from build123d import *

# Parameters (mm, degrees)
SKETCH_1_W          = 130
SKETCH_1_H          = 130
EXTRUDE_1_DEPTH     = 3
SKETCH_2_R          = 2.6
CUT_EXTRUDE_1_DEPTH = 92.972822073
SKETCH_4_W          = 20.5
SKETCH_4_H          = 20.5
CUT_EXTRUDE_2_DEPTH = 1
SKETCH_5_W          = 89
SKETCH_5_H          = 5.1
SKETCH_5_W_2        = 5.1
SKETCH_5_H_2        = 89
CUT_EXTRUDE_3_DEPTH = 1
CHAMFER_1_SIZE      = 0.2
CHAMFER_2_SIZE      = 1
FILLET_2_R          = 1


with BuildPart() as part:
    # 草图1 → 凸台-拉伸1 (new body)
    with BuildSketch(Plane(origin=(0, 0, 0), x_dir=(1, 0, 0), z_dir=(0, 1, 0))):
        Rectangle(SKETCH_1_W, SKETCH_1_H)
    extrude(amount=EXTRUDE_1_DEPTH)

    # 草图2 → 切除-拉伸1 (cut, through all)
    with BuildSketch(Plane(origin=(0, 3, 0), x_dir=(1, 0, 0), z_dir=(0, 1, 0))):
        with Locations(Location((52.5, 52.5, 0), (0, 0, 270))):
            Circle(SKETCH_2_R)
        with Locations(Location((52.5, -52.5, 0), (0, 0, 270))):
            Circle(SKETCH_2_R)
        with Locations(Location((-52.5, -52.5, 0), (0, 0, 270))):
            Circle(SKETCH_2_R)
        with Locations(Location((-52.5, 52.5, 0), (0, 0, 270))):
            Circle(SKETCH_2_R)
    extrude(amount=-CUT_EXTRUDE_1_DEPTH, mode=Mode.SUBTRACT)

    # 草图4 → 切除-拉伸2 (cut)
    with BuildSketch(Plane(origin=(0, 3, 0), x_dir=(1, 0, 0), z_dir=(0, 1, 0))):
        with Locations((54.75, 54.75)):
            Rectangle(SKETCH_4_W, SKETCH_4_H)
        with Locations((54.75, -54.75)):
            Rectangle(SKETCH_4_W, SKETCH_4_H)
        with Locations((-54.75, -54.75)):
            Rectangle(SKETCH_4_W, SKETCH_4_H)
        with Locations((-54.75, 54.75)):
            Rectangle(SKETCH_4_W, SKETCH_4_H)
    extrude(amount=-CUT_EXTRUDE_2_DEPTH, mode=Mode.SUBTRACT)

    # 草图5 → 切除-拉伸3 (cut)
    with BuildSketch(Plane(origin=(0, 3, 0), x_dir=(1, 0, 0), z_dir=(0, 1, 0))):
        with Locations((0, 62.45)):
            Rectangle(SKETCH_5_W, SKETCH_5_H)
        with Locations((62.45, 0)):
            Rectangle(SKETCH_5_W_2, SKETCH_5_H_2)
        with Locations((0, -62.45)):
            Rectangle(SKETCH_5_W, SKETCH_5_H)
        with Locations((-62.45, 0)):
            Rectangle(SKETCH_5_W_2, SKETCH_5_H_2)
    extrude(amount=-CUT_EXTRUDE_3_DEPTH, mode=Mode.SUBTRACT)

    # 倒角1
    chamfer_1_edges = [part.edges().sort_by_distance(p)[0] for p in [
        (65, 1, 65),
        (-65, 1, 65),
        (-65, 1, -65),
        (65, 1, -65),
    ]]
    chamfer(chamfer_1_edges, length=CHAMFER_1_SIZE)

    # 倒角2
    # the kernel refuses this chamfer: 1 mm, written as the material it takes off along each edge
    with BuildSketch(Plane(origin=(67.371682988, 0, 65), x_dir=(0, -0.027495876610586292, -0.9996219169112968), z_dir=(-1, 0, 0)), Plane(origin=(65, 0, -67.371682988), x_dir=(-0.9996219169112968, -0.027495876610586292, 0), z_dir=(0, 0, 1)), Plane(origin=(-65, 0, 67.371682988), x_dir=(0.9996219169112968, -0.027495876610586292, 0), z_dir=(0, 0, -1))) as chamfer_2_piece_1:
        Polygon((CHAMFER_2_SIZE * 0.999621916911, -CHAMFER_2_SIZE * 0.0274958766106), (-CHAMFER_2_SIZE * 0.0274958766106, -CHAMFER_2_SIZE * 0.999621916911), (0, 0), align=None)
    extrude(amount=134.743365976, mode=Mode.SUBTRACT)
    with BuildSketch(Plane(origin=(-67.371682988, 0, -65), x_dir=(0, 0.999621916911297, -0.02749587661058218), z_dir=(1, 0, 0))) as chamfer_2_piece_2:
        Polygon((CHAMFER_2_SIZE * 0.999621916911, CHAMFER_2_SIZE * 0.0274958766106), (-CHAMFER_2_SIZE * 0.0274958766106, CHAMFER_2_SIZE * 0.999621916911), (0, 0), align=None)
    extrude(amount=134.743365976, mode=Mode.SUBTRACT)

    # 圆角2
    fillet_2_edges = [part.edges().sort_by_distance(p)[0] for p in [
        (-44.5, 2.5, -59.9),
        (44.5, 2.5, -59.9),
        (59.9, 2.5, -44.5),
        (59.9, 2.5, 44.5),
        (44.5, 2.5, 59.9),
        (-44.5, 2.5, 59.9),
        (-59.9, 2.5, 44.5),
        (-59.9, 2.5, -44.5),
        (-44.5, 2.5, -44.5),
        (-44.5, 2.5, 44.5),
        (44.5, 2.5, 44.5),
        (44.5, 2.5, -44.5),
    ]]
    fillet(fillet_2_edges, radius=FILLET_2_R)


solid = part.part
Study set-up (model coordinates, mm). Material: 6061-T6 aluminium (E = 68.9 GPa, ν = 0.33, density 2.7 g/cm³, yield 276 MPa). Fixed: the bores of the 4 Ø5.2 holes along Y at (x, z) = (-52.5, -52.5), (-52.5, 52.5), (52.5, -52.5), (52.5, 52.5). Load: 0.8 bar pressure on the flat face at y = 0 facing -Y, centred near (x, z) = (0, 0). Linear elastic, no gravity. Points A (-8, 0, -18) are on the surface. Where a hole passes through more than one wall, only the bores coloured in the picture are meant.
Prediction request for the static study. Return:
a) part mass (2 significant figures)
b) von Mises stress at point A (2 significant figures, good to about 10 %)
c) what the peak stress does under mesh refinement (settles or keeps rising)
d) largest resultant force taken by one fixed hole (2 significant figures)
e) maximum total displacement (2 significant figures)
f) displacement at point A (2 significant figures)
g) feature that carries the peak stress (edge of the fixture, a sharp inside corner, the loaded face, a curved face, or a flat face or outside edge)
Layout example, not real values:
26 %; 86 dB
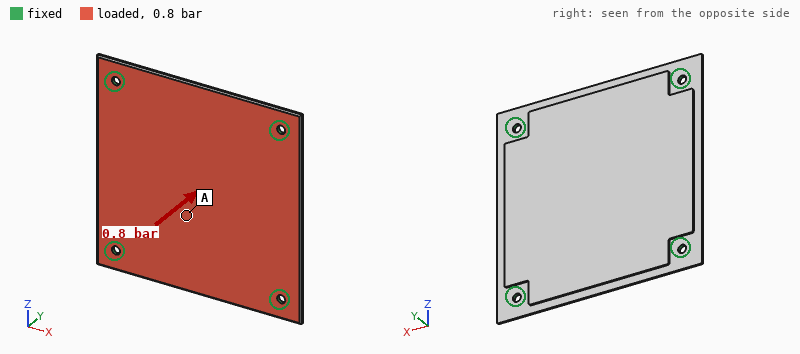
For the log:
130 g; 33 MPa; keeps rising; 790 N; 0.57 mm; 0.53 mm; edge of the fixture
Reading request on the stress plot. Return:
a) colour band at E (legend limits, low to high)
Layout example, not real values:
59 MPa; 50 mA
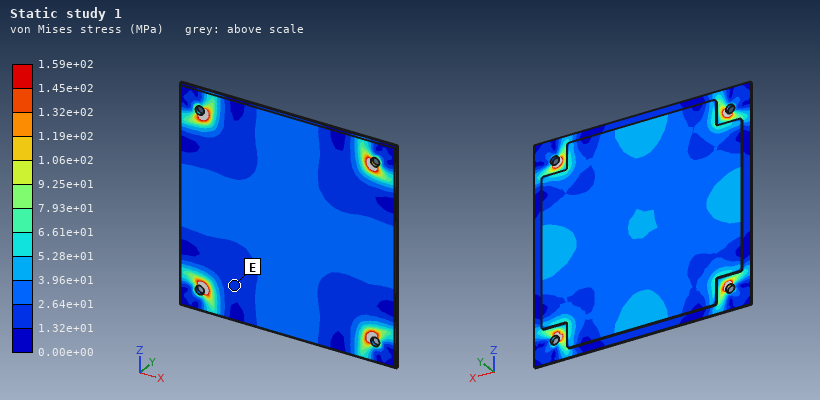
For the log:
1.32e+01 to 2.64e+01 MPa
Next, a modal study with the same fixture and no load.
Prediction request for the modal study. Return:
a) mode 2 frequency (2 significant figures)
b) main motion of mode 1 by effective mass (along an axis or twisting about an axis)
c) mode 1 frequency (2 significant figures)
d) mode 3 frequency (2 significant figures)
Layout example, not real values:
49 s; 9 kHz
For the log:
1300 Hz; along Y; 800 Hz; 1300 Hz
